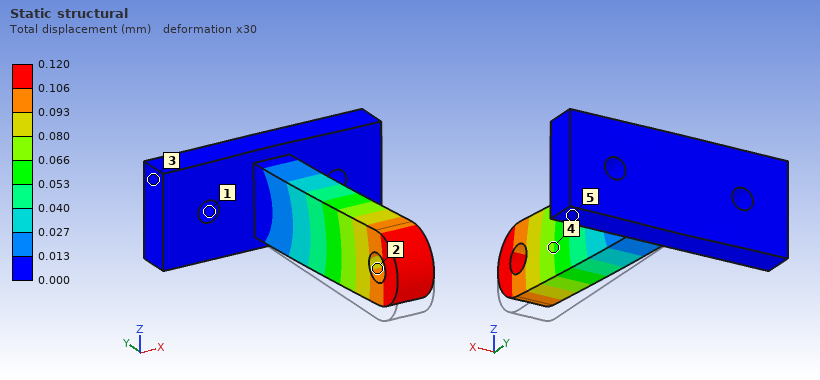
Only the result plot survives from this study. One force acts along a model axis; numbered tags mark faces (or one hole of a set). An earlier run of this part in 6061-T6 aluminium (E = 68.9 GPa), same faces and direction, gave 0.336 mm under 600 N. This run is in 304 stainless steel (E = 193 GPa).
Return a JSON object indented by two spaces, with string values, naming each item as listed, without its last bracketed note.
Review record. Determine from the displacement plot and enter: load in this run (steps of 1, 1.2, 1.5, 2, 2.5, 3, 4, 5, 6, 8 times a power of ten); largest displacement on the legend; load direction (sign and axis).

{
  "load in this run": "600 N",
  "largest displacement on the legend": "0.120 mm",
  "load direction": "+Z"
}
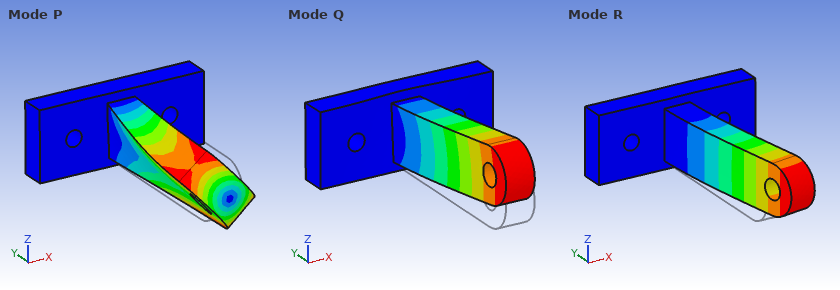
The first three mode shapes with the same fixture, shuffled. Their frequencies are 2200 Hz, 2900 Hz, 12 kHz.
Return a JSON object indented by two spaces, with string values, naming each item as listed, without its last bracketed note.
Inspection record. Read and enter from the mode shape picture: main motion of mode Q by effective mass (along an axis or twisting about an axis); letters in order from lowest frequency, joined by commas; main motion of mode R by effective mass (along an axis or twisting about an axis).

{
  "main motion of mode Q by effective mass": "along Z",
  "letters in order from lowest frequency, joined by commas": "R, Q, P",
  "main motion of mode R by effective mass": "along X"
}
